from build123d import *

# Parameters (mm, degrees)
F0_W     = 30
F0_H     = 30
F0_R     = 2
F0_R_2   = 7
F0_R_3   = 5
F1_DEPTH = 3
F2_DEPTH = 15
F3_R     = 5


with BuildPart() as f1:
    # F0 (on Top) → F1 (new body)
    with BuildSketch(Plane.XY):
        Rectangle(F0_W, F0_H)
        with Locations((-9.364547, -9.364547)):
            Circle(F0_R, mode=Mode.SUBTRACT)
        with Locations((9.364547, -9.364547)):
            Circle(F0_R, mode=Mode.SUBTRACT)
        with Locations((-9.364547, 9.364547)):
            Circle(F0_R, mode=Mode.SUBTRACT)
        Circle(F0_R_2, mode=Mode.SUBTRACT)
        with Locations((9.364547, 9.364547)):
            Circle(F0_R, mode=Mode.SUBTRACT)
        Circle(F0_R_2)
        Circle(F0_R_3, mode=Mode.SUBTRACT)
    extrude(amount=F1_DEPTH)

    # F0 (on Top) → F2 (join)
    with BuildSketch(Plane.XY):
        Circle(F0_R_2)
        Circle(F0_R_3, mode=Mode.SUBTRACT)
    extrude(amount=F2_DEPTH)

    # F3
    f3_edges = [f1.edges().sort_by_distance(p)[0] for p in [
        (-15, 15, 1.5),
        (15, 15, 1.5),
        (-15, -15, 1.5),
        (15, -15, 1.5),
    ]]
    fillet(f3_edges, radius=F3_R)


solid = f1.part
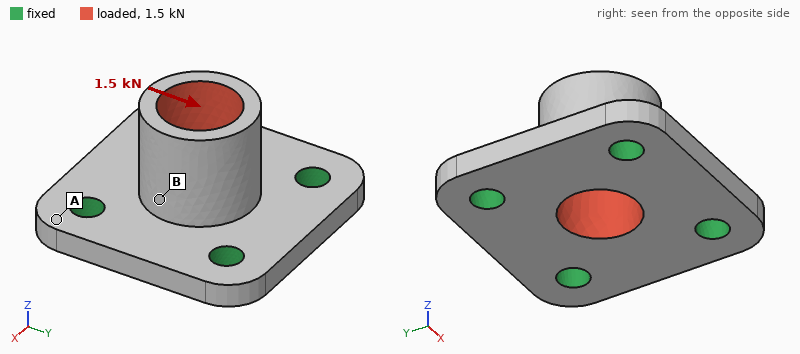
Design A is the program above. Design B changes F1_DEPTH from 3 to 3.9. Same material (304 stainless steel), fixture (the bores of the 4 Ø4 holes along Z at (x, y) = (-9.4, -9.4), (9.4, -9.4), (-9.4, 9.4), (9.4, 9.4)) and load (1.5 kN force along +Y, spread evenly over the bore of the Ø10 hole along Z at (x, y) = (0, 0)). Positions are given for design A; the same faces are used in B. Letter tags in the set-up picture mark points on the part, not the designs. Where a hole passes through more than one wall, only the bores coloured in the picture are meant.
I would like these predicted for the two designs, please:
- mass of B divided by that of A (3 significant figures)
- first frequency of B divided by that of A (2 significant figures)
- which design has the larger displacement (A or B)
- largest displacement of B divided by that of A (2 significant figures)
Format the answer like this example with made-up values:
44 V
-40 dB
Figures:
1.19
1.2
A
0.66
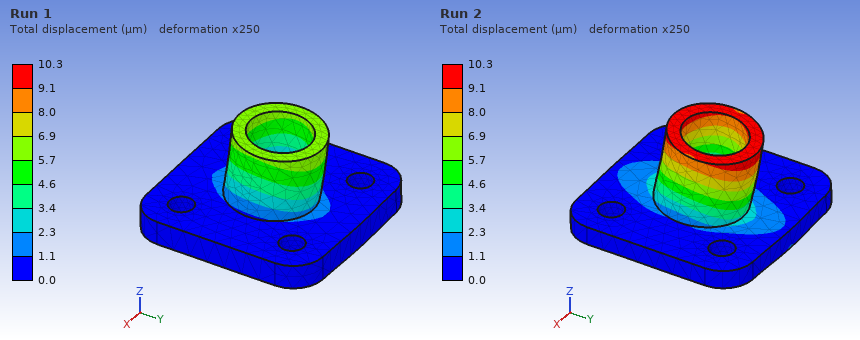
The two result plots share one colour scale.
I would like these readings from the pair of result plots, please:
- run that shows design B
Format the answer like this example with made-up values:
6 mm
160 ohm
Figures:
Run 1
